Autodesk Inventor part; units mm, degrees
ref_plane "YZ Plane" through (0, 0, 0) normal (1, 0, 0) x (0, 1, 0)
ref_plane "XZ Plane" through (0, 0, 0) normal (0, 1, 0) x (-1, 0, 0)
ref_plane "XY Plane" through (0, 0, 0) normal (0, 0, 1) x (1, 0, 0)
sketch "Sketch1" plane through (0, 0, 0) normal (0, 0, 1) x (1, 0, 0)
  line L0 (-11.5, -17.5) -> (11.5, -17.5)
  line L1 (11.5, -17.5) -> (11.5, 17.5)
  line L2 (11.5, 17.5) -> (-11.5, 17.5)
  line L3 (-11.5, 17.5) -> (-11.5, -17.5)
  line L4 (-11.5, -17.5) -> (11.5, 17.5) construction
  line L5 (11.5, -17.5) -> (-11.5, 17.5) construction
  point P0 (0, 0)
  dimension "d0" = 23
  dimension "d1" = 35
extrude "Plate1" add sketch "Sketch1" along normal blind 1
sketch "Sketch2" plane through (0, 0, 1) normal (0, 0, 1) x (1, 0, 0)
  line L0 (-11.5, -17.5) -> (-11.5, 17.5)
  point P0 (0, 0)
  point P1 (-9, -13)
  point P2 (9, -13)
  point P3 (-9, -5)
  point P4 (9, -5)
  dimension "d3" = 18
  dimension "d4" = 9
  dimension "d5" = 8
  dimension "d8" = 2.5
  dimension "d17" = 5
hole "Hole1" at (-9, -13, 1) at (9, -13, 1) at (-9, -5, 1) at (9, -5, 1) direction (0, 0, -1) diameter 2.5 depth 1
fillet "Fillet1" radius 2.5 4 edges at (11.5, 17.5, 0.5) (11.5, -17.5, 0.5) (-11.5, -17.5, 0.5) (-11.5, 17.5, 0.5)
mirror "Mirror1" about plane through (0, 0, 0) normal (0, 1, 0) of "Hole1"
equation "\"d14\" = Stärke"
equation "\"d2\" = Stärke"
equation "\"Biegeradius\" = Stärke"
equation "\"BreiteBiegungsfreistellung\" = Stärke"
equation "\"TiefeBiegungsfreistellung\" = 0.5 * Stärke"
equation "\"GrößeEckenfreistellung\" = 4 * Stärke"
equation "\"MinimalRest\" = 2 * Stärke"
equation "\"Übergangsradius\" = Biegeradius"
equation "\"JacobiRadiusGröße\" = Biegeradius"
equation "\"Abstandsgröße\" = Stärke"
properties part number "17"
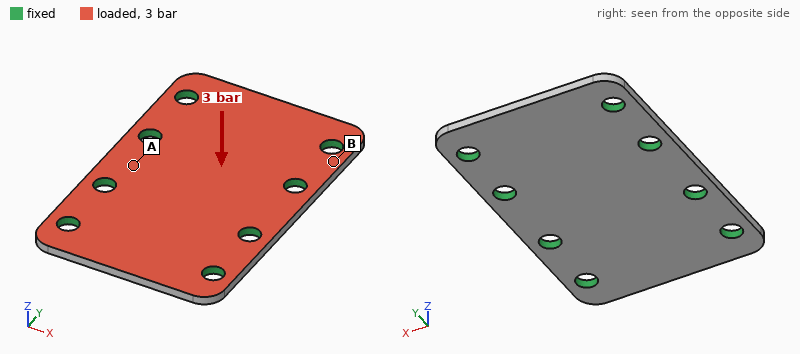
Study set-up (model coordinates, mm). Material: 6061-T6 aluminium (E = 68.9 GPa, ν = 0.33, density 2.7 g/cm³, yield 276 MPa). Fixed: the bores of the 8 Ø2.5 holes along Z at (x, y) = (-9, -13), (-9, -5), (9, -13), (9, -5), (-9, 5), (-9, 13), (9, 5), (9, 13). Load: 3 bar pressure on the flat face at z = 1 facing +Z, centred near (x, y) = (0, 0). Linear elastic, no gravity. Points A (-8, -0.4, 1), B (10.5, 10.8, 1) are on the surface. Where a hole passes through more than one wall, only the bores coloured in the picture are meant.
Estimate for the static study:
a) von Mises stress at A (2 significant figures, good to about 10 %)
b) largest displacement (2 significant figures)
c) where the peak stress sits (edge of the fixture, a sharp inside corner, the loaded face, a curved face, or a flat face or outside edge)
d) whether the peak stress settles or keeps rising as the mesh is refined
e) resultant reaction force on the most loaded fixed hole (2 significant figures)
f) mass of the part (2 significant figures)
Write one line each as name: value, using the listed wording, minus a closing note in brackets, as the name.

von Mises stress at A: 14 MPa
largest displacement: 14 µm
where the peak stress sits: edge of the fixture
whether the peak stress settles or keeps rising as the mesh is refined: keeps rising
resultant reaction force on the most loaded fixed hole: 29 N
mass of the part: 2.1 g
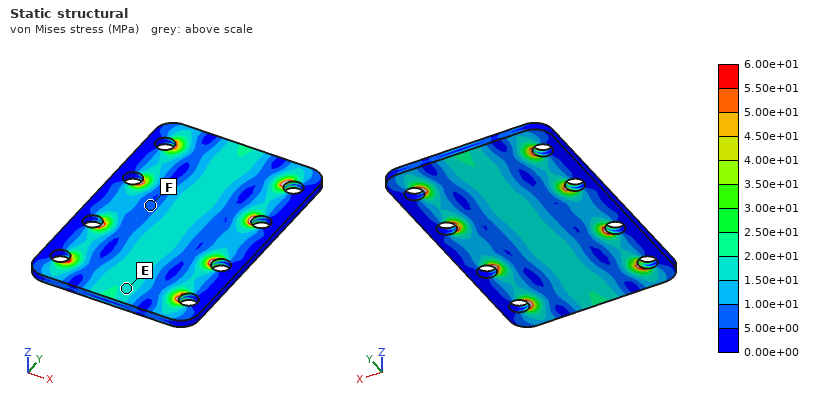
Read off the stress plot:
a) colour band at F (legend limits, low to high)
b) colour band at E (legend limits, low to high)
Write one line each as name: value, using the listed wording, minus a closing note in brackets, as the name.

colour band at F: 5.00e+00 to 1.00e+01 MPa
colour band at E: 1.50e+01 to 2.00e+01 MPa
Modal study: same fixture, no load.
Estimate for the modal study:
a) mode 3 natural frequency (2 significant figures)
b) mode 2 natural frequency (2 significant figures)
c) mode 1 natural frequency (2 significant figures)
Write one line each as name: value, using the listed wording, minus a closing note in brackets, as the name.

mode 3 natural frequency: 21 kHz
mode 2 natural frequency: 19 kHz
mode 1 natural frequency: 18 kHz
